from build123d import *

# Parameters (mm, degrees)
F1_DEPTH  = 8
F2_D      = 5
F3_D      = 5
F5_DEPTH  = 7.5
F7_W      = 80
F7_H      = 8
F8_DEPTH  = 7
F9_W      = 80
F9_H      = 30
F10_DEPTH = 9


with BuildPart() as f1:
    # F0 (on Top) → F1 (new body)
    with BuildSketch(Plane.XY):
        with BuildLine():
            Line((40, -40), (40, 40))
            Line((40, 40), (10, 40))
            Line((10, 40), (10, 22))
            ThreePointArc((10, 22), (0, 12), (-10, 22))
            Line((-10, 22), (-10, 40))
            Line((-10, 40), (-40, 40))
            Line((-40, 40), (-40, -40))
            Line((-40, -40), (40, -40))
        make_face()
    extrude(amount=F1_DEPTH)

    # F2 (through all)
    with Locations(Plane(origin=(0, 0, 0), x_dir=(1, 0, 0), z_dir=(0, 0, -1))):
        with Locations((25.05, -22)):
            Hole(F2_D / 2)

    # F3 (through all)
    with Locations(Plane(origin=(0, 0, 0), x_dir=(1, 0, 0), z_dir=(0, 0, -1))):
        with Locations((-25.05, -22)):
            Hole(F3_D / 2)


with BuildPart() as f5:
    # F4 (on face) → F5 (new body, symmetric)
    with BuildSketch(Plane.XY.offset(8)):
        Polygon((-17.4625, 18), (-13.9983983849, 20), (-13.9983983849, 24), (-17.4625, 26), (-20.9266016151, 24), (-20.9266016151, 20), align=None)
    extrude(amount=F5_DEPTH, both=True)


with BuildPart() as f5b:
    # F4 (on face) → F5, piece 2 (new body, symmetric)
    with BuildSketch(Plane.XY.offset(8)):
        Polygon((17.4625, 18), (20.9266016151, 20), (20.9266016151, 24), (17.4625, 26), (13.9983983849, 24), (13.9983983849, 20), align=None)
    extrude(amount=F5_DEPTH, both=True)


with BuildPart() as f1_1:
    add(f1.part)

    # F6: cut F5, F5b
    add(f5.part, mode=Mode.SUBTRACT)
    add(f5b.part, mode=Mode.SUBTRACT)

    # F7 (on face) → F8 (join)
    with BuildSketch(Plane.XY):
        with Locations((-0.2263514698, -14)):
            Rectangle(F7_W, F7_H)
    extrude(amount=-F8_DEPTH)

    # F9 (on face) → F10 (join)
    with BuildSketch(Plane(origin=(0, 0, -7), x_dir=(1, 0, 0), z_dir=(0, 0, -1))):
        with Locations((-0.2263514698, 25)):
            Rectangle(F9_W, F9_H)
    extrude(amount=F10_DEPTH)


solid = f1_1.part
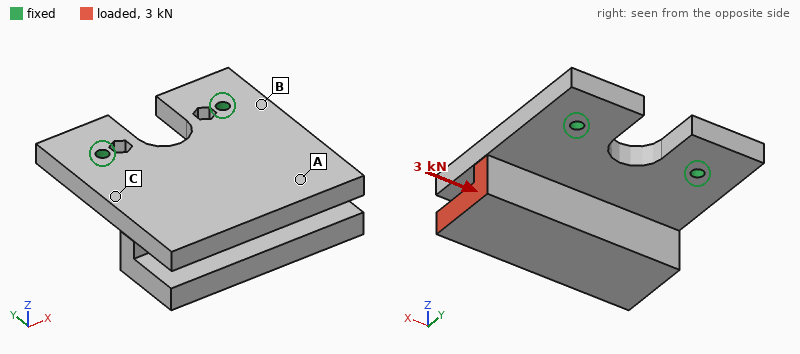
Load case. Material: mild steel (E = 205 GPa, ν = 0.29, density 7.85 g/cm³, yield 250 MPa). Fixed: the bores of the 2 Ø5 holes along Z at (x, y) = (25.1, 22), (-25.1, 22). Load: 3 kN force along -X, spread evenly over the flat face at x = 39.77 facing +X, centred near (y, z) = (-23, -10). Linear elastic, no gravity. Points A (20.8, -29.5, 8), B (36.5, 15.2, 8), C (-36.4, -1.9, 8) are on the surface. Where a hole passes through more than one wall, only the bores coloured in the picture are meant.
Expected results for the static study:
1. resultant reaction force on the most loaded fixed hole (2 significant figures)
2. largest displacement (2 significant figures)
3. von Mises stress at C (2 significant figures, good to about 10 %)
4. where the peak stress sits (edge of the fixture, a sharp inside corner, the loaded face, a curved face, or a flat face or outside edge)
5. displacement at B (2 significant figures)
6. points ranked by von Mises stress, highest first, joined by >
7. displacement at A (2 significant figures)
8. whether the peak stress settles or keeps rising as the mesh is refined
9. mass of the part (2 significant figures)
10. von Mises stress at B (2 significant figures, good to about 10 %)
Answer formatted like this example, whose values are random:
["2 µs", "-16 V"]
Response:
["2.9 kN", "27 µm", "14 MPa", "edge of the fixture", "5.3 µm", "B > C > A", "12 µm", "keeps rising", "570 g", "26 MPa"]
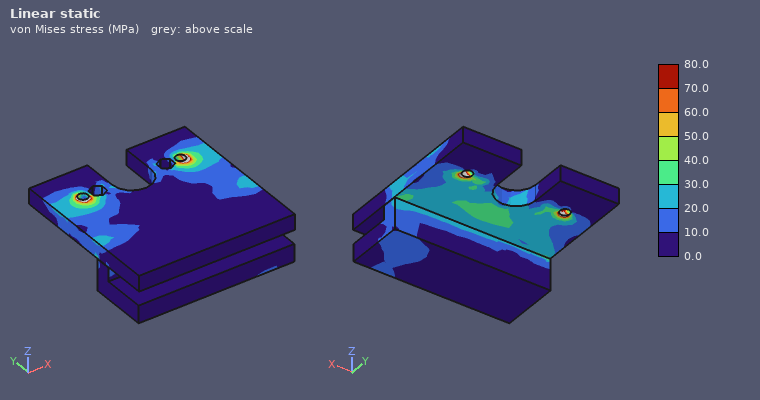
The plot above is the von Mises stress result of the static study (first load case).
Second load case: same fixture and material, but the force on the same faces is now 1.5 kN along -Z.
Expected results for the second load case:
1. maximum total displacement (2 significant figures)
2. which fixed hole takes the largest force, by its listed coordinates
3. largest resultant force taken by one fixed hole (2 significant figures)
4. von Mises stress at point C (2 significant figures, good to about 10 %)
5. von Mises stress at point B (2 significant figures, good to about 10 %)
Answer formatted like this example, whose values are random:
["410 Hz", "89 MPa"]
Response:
["0.21 mm", "(25.1, 22)", "1.7 kN", "52 MPa", "100 MPa"]
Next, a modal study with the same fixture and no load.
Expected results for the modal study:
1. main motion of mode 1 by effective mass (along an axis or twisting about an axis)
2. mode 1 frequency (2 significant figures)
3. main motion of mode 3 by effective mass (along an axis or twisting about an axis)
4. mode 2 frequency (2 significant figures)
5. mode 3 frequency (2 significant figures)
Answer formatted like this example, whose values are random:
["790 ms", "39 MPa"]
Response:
["along Z", "950 Hz", "along X", "2500 Hz", "4900 Hz"]
